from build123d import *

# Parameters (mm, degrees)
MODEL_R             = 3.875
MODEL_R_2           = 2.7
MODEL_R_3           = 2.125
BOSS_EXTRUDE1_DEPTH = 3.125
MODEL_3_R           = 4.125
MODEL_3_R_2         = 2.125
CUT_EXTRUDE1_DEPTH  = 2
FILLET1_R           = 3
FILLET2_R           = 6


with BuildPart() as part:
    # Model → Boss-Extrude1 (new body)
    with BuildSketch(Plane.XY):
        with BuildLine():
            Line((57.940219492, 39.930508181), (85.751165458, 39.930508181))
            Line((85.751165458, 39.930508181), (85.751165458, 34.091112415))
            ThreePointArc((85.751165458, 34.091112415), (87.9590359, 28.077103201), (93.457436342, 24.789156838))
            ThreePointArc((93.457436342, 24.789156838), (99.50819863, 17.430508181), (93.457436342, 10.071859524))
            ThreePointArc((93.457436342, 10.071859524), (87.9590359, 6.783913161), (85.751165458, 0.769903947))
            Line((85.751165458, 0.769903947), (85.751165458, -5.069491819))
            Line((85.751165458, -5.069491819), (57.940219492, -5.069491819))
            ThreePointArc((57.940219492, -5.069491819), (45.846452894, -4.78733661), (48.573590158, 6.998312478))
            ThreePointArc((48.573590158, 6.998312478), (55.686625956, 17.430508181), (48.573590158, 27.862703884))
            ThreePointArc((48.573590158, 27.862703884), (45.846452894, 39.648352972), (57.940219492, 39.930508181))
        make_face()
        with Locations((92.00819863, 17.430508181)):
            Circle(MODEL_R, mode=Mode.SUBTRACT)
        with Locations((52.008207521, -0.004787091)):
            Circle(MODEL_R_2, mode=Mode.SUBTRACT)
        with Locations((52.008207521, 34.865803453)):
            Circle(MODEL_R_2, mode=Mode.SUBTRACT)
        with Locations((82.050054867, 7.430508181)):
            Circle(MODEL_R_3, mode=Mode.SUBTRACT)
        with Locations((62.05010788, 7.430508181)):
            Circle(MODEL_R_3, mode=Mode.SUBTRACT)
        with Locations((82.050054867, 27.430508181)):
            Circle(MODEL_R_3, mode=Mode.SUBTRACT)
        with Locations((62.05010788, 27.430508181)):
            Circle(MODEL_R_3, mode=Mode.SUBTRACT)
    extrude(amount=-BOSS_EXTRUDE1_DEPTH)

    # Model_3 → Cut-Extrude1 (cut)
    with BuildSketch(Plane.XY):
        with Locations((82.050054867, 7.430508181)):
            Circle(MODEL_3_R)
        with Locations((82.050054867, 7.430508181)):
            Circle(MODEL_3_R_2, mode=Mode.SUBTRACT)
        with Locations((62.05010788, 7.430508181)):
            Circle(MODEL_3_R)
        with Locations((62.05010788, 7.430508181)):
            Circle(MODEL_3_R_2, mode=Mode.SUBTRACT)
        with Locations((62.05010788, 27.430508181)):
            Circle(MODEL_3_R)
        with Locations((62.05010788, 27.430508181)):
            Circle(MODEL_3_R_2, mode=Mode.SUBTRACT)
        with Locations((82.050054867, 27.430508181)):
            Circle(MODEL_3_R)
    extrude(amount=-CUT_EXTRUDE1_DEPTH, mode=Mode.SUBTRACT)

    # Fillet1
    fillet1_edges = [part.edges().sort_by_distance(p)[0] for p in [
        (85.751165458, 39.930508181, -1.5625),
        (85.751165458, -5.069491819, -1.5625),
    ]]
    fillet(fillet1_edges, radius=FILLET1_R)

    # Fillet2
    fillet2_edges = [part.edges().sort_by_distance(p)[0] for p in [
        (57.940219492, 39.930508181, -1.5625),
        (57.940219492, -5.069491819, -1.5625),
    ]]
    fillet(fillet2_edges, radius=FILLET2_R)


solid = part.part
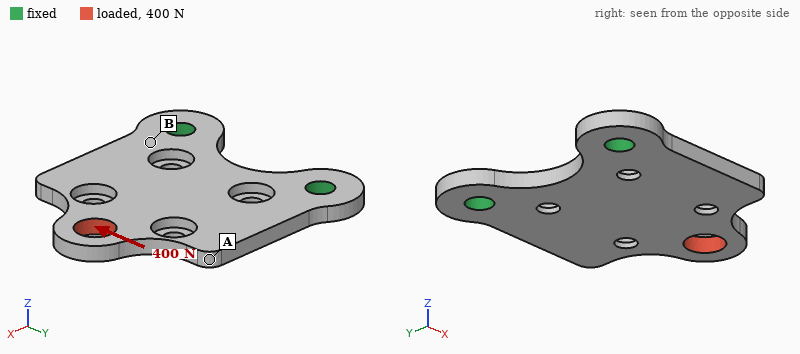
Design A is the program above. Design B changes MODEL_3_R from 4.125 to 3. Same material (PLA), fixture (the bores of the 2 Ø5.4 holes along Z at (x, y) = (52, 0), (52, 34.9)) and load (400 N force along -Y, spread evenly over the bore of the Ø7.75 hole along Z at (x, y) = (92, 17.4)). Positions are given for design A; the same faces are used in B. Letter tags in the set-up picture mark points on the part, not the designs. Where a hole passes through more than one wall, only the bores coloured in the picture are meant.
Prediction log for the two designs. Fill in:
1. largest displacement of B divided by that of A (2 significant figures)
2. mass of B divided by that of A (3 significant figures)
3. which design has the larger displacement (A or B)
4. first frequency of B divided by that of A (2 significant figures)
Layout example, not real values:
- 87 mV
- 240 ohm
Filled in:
- 0.90
- 1.04
- A
- 1.0
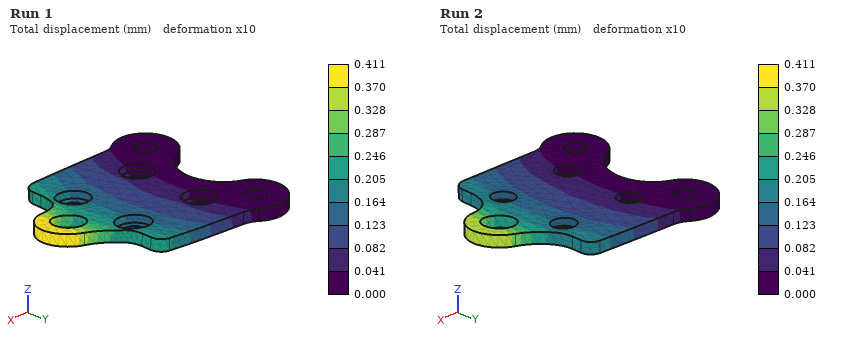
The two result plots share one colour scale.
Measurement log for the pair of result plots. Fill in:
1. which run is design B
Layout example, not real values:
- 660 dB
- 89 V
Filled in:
- Run 2
